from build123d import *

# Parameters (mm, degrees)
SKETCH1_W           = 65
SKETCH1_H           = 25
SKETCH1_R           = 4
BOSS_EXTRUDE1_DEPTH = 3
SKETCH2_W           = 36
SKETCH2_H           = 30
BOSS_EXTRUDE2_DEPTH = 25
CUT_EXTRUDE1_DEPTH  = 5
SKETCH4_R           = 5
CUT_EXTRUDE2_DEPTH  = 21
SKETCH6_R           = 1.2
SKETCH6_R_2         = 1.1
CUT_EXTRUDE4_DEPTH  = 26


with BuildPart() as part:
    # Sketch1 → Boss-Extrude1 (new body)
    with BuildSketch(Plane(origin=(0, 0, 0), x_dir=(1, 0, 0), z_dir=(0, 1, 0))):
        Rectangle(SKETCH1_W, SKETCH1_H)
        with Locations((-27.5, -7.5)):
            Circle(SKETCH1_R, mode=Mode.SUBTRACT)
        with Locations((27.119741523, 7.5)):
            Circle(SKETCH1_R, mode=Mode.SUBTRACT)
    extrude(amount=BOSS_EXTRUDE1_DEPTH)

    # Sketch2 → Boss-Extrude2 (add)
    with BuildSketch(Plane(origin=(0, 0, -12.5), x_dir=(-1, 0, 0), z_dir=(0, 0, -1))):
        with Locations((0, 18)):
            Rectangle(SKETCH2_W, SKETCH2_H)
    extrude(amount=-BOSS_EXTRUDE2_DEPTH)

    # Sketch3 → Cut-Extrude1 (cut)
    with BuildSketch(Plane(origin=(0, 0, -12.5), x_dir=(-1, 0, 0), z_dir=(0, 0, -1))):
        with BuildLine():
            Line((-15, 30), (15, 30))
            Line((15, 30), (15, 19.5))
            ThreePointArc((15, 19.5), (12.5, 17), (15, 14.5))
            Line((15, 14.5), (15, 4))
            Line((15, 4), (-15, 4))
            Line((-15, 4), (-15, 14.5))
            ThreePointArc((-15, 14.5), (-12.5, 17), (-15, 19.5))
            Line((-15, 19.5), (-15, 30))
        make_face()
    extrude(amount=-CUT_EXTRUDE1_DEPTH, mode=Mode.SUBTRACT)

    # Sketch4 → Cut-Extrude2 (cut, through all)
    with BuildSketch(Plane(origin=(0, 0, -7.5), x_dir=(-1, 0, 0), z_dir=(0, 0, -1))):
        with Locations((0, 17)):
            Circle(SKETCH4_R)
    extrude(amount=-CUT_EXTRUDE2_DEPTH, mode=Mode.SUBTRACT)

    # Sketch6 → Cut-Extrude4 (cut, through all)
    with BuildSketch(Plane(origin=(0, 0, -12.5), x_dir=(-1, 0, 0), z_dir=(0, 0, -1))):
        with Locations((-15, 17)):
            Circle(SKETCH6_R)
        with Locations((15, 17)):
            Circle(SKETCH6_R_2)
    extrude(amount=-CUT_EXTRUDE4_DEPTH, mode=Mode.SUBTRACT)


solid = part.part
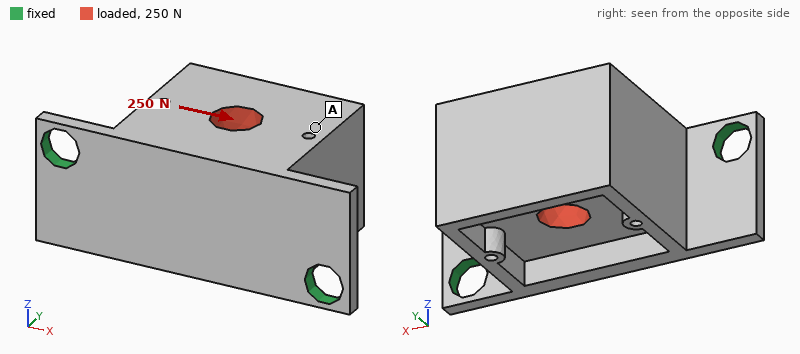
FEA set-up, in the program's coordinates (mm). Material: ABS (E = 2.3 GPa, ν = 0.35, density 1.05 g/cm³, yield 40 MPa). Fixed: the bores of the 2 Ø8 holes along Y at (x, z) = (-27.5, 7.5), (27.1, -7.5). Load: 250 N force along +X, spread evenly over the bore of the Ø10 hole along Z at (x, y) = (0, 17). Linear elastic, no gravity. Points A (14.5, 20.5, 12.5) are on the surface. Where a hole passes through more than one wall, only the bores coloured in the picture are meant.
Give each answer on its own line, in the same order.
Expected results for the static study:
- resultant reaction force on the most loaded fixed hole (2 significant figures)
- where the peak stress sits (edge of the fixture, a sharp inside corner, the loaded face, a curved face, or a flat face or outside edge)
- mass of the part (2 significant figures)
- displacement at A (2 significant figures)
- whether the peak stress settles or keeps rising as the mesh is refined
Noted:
150 N
edge of the fixture
27 g
0.42 mm
keeps rising
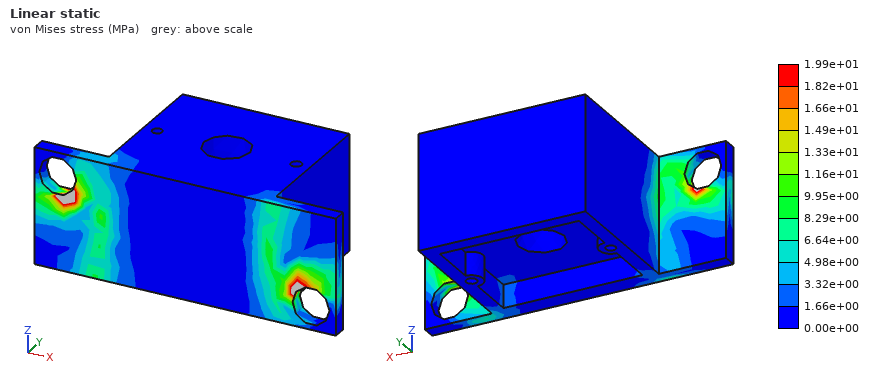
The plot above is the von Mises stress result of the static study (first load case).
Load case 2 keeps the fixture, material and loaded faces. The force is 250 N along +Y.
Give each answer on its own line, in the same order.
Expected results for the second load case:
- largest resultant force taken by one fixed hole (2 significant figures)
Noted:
150 N
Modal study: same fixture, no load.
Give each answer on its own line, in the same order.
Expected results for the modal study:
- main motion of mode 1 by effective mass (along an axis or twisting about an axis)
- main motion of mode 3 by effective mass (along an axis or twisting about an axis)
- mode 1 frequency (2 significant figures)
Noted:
along Z
along X
420 Hz
